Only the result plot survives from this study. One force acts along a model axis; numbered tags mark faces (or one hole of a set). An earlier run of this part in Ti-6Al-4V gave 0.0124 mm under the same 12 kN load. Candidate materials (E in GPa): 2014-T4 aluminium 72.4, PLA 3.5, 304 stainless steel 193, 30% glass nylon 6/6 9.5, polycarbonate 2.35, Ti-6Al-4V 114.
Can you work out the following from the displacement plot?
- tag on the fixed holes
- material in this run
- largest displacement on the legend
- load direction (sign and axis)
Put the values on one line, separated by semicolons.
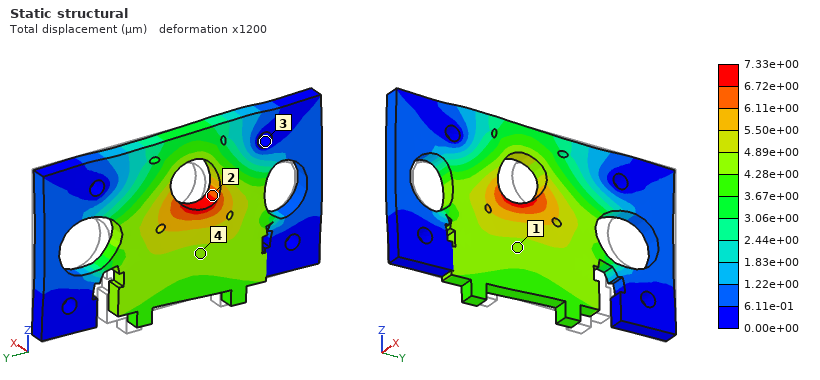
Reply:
3; 304 stainless steel; 7.33e+00 µm; -Y
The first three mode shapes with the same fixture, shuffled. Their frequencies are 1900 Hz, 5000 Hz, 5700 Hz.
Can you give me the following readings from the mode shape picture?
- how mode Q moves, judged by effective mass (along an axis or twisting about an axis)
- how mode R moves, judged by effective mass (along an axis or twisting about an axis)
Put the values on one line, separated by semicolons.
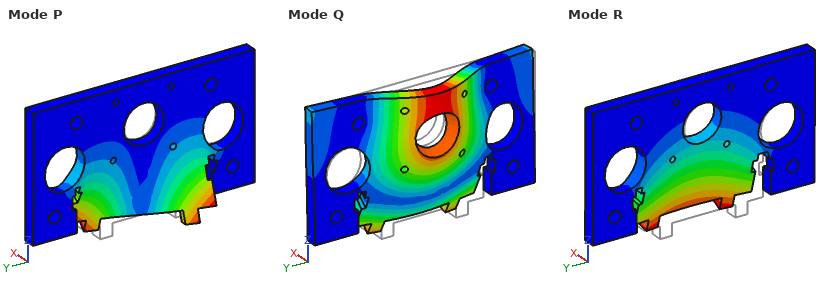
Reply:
along X; along X
